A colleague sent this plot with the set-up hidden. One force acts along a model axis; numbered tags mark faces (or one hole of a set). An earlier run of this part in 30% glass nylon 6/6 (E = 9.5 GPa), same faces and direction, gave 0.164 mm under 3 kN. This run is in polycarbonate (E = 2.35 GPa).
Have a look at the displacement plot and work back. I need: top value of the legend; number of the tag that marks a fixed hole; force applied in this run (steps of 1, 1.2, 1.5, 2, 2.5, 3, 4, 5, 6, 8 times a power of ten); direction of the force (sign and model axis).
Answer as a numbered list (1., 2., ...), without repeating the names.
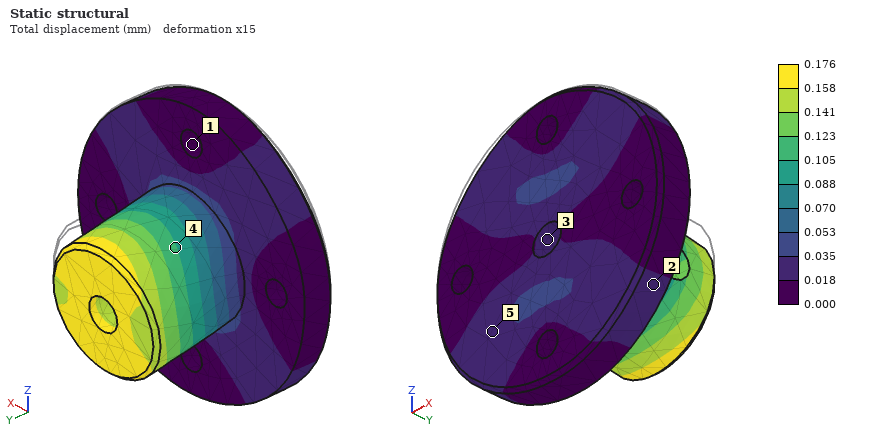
1. 0.176 mm
2. 1
3. 800 N
4. -Z
